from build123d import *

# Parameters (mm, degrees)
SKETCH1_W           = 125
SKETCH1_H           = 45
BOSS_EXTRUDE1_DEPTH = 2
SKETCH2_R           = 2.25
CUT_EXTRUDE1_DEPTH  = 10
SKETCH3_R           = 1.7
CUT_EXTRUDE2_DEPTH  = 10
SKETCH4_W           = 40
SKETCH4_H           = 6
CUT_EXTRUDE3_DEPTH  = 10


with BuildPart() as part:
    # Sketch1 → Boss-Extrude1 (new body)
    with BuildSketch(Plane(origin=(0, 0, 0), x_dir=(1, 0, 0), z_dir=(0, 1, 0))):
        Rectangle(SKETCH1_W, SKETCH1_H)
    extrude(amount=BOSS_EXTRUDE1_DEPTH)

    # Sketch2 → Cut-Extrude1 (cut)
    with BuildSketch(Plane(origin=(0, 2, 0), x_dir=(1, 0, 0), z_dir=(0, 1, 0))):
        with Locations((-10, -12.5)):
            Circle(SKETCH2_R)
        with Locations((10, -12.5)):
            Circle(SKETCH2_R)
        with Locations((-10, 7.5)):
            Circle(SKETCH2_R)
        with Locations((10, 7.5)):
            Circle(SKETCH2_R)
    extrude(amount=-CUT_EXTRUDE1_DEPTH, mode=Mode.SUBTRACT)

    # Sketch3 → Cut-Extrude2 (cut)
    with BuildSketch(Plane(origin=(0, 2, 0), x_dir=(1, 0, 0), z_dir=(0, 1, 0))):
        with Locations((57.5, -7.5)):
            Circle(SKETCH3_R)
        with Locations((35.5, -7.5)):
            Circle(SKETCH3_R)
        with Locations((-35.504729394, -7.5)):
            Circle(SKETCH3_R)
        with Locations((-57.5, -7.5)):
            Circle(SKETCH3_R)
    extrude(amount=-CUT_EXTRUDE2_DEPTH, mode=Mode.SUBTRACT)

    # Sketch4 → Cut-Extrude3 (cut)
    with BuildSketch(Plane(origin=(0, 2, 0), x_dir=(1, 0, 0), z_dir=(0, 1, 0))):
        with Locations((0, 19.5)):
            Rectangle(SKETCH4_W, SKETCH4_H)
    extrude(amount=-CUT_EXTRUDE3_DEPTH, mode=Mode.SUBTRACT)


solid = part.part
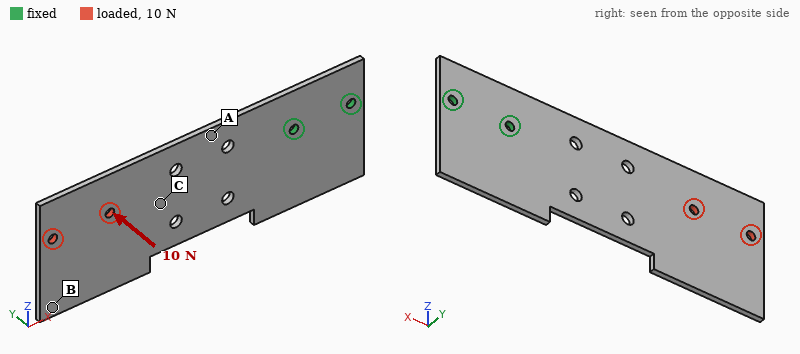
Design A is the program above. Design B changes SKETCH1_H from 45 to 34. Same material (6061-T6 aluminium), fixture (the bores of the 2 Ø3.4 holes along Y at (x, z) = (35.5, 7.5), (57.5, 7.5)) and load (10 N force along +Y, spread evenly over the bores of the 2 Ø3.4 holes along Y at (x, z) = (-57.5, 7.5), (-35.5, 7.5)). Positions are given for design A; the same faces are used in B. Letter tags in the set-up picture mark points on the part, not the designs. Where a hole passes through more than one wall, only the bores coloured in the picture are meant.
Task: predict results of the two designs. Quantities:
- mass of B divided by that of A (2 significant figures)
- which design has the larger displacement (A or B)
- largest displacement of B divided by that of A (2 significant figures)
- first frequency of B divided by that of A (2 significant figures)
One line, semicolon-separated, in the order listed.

0.78; B; 1.2; 1.0
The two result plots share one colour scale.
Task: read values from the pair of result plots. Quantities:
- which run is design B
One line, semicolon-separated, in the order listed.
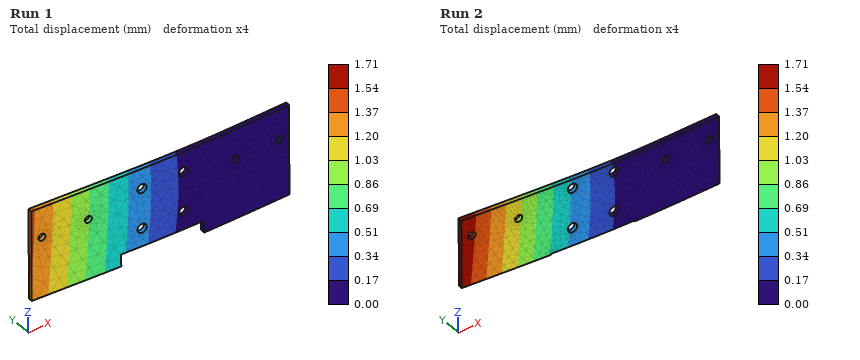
Run 2
